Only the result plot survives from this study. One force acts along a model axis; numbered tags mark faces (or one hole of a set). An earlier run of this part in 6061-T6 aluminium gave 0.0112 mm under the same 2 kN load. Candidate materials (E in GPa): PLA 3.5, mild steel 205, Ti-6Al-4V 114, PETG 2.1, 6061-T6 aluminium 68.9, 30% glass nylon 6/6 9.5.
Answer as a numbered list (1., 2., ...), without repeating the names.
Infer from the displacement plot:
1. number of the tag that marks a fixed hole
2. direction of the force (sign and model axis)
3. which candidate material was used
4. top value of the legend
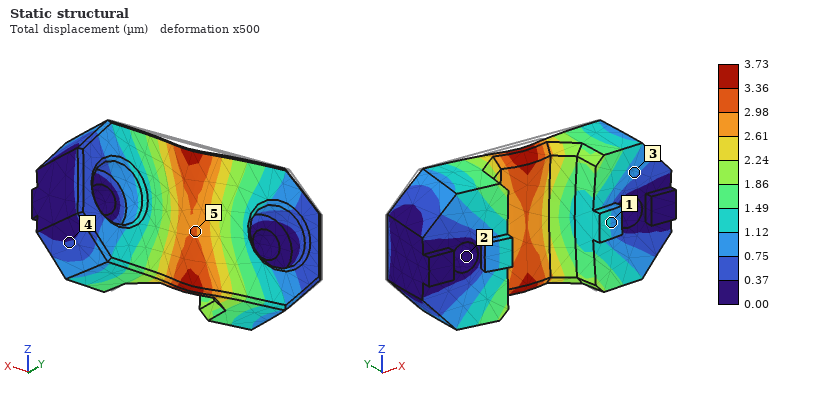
1. 2
2. -Y
3. mild steel
4. 3.73 µm
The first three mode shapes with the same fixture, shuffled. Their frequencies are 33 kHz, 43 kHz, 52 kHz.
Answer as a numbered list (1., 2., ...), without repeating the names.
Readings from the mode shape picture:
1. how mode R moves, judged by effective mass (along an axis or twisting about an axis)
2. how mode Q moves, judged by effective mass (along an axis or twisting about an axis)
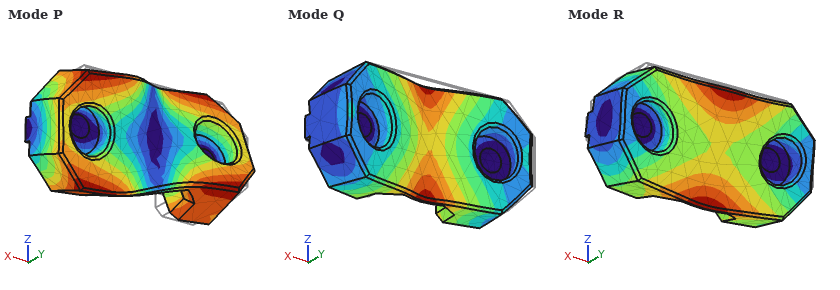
1. along Z
2. along Y
